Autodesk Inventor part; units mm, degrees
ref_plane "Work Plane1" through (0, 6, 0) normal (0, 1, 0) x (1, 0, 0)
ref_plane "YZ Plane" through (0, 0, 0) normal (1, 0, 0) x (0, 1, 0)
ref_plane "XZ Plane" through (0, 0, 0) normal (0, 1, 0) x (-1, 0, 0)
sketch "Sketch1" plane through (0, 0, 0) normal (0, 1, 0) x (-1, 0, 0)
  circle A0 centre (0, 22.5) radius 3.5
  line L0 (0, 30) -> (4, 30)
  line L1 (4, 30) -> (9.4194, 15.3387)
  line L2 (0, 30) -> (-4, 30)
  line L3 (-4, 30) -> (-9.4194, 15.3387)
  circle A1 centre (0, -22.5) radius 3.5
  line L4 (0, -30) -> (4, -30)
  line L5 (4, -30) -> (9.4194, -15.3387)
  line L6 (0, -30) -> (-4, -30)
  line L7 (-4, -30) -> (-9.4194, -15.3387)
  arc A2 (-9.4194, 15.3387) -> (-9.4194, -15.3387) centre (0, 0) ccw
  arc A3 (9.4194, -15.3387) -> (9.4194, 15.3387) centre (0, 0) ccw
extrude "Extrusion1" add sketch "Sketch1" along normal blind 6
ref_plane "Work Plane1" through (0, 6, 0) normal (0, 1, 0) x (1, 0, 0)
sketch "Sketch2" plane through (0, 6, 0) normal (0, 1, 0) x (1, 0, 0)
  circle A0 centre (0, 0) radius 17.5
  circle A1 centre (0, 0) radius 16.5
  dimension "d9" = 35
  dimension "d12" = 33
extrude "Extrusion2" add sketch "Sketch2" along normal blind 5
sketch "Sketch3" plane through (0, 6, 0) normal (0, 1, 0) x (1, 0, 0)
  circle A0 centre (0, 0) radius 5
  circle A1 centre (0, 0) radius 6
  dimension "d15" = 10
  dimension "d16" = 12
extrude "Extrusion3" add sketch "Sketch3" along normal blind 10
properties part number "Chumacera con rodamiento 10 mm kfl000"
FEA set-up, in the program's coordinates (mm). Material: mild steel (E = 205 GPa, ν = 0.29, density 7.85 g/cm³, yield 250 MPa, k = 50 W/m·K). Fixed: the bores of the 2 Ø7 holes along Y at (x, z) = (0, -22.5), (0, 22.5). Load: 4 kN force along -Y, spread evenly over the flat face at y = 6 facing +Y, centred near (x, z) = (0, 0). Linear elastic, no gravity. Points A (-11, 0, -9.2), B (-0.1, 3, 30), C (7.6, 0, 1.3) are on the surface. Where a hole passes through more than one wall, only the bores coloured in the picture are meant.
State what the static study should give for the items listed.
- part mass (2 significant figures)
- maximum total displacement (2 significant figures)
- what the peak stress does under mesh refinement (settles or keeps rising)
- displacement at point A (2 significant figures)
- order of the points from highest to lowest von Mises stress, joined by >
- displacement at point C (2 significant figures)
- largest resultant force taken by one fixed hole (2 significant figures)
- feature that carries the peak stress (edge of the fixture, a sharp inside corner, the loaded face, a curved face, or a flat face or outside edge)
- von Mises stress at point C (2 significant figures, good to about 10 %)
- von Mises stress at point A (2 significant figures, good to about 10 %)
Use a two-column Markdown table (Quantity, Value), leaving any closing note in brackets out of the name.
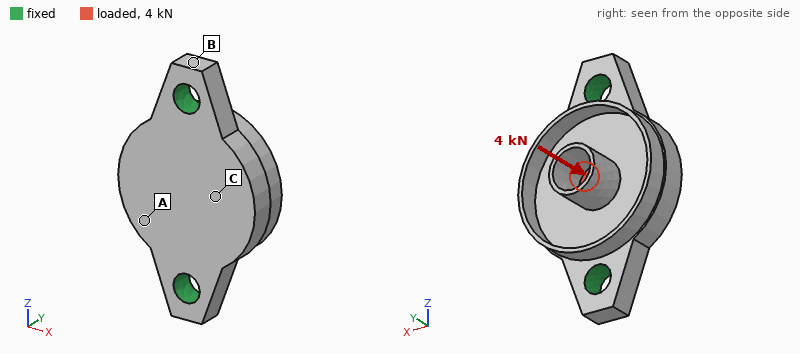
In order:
| Quantity | Value |
|---|---|
| part mass | 67 g |
| maximum total displacement | 20 µm |
| what the peak stress does under mesh refinement | keeps rising |
| displacement at point A | 12 µm |
| order of the points from highest to lowest von Mises stress, joined by > | C > A > B |
| displacement at point C | 17 µm |
| largest resultant force taken by one fixed hole | 2.0 kN |
| feature that carries the peak stress | edge of the fixture |
| von Mises stress at point C | 74 MPa |
| von Mises stress at point A | 43 MPa |
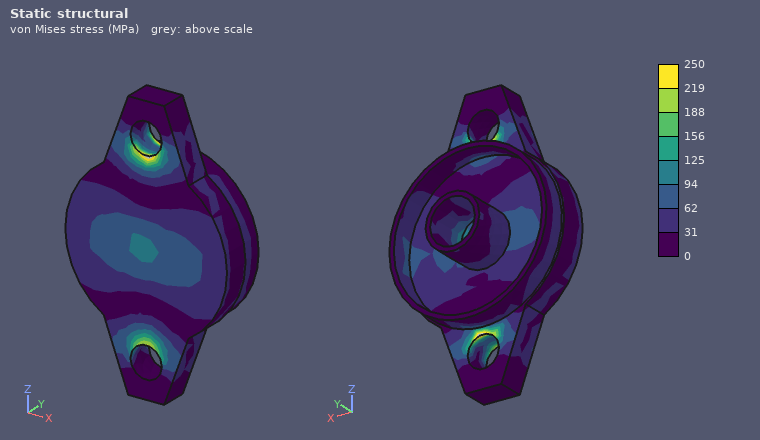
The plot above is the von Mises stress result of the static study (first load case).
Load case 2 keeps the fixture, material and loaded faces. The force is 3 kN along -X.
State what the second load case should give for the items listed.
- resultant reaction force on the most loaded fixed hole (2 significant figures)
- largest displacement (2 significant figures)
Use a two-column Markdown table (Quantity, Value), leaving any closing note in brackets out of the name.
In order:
| Quantity | Value |
|---|---|
| resultant reaction force on the most loaded fixed hole | 1.5 kN |
| largest displacement | 11 µm |
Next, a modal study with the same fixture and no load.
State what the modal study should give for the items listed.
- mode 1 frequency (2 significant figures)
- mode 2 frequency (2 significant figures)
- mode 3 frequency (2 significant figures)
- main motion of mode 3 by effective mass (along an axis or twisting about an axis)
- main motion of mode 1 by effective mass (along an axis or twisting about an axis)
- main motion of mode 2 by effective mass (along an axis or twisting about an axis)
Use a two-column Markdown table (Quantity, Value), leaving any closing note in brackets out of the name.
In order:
| Quantity | Value |
|---|---|
| mode 1 frequency | 10 kHz |
| mode 2 frequency | 12 kHz |
| mode 3 frequency | 25 kHz |
| main motion of mode 3 by effective mass | along X |
| main motion of mode 1 by effective mass | twisting about Z |
| main motion of mode 2 by effective mass | along Y |
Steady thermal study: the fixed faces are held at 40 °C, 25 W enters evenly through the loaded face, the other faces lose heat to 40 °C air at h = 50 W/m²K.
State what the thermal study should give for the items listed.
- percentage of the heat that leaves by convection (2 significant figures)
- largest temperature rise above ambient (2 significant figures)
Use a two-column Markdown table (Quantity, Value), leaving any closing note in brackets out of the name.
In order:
| Quantity | Value |
|---|---|
| percentage of the heat that leaves by convection | 18 % |
| largest temperature rise above ambient | 49 K |
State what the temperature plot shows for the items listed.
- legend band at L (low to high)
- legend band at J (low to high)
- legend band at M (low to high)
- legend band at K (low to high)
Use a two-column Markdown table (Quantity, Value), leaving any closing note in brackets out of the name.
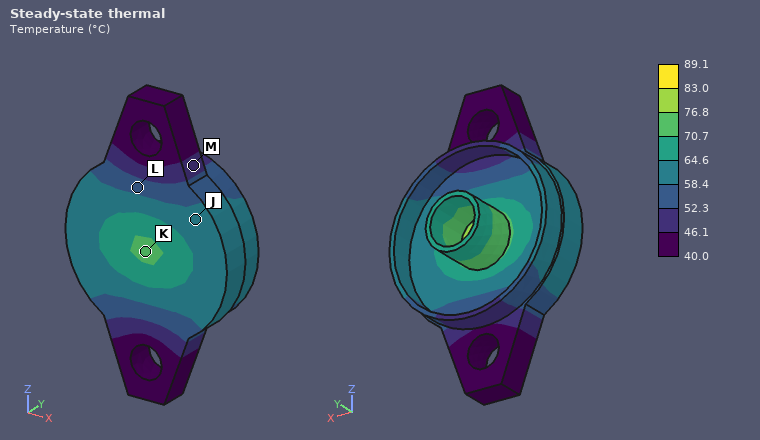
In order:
| Quantity | Value |
|---|---|
| legend band at L | 52.3 to 58.4 °C |
| legend band at J | 58.4 to 64.6 °C |
| legend band at M | 46.1 to 52.3 °C |
| legend band at K | 70.7 to 76.8 °C |
